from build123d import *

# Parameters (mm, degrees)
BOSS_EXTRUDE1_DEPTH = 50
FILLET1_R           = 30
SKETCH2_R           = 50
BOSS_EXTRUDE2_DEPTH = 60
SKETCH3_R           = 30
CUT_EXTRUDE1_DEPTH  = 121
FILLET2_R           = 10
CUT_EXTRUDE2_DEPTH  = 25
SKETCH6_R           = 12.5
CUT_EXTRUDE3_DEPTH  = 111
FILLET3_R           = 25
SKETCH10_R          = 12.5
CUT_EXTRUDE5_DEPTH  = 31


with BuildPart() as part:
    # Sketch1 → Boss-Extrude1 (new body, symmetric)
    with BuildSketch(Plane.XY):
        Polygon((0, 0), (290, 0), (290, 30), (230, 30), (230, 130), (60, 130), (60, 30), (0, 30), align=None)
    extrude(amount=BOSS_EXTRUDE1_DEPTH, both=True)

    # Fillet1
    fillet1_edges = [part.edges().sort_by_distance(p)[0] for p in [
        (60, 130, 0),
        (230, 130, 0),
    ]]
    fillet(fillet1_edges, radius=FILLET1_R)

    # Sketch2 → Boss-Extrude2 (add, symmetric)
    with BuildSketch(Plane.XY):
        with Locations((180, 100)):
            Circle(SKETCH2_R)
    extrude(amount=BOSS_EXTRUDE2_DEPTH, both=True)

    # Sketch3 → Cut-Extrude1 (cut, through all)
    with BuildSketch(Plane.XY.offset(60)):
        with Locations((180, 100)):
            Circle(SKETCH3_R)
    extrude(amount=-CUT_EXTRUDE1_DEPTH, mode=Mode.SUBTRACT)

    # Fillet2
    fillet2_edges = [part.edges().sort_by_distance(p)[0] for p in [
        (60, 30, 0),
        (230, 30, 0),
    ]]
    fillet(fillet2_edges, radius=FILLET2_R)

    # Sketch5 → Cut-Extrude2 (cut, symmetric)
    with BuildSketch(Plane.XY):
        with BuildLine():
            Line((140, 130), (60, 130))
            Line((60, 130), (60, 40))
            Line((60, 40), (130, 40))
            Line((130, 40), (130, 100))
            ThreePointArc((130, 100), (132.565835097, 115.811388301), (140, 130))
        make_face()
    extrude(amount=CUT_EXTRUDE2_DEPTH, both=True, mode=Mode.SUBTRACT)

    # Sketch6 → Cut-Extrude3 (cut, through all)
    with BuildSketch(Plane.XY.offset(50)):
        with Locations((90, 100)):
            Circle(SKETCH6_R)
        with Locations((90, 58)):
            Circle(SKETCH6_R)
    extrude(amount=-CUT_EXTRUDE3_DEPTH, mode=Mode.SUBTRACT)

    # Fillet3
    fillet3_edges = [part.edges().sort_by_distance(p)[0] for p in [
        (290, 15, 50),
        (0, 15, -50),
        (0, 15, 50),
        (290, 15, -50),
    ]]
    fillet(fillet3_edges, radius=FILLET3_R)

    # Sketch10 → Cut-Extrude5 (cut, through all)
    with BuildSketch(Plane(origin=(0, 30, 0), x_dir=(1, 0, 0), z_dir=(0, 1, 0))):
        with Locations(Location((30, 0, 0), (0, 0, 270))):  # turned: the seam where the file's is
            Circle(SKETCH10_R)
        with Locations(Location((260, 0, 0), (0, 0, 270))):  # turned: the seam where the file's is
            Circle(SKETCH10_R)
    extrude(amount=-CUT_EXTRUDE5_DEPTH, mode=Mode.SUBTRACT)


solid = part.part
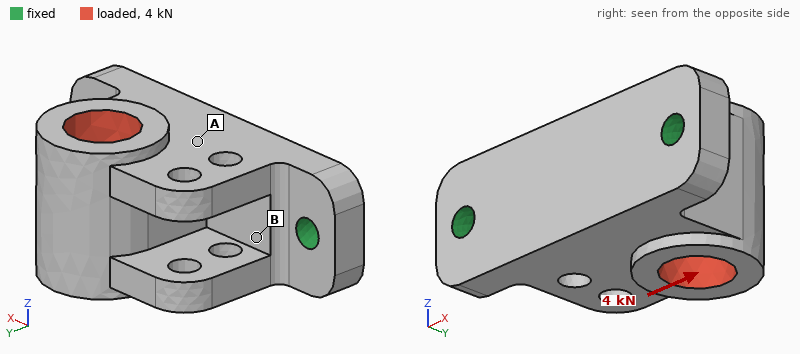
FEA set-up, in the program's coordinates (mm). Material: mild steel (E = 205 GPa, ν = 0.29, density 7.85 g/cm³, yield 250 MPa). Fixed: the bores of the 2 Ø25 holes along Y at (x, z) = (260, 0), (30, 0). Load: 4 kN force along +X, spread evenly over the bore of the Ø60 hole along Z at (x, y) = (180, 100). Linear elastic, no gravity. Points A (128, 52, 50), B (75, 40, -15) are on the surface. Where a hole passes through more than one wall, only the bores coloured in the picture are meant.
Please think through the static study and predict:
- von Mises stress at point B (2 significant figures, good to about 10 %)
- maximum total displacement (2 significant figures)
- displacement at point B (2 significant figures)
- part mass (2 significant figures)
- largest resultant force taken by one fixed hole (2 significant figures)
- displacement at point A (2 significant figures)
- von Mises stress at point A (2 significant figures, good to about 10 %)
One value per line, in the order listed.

1.5 MPa
2.1 µm
0.48 µm
16 kg
2.6 kN
0.64 µm
0.63 MPa
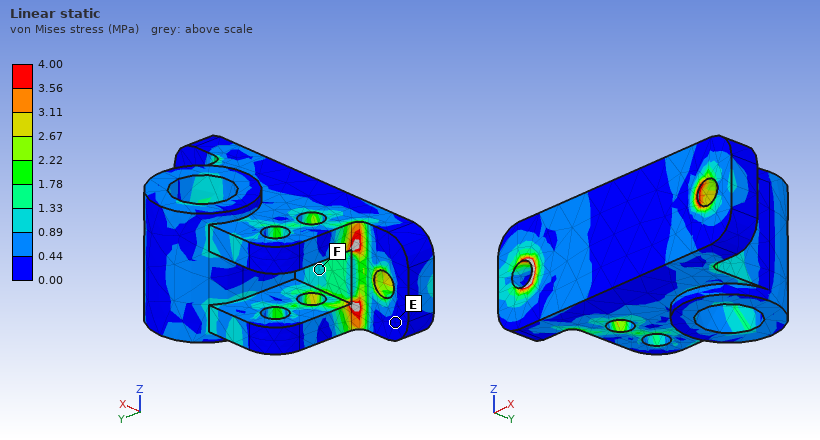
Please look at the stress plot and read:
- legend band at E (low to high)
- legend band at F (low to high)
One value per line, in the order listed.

0.00 to 0.44 MPa
0.89 to 1.33 MPa
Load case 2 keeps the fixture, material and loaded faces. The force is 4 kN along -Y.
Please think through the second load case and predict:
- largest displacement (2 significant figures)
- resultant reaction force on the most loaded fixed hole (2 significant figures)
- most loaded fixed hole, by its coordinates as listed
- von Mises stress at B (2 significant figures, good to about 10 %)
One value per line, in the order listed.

1.3 µm
2.9 kN
(260, 0)
0.86 MPa
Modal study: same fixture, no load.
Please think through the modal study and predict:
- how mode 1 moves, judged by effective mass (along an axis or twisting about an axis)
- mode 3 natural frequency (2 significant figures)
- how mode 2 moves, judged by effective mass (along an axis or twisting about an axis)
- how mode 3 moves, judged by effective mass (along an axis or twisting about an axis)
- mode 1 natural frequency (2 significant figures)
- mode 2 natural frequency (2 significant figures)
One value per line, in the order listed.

along Z
3100 Hz
along Y
along X
1100 Hz
2600 Hz
